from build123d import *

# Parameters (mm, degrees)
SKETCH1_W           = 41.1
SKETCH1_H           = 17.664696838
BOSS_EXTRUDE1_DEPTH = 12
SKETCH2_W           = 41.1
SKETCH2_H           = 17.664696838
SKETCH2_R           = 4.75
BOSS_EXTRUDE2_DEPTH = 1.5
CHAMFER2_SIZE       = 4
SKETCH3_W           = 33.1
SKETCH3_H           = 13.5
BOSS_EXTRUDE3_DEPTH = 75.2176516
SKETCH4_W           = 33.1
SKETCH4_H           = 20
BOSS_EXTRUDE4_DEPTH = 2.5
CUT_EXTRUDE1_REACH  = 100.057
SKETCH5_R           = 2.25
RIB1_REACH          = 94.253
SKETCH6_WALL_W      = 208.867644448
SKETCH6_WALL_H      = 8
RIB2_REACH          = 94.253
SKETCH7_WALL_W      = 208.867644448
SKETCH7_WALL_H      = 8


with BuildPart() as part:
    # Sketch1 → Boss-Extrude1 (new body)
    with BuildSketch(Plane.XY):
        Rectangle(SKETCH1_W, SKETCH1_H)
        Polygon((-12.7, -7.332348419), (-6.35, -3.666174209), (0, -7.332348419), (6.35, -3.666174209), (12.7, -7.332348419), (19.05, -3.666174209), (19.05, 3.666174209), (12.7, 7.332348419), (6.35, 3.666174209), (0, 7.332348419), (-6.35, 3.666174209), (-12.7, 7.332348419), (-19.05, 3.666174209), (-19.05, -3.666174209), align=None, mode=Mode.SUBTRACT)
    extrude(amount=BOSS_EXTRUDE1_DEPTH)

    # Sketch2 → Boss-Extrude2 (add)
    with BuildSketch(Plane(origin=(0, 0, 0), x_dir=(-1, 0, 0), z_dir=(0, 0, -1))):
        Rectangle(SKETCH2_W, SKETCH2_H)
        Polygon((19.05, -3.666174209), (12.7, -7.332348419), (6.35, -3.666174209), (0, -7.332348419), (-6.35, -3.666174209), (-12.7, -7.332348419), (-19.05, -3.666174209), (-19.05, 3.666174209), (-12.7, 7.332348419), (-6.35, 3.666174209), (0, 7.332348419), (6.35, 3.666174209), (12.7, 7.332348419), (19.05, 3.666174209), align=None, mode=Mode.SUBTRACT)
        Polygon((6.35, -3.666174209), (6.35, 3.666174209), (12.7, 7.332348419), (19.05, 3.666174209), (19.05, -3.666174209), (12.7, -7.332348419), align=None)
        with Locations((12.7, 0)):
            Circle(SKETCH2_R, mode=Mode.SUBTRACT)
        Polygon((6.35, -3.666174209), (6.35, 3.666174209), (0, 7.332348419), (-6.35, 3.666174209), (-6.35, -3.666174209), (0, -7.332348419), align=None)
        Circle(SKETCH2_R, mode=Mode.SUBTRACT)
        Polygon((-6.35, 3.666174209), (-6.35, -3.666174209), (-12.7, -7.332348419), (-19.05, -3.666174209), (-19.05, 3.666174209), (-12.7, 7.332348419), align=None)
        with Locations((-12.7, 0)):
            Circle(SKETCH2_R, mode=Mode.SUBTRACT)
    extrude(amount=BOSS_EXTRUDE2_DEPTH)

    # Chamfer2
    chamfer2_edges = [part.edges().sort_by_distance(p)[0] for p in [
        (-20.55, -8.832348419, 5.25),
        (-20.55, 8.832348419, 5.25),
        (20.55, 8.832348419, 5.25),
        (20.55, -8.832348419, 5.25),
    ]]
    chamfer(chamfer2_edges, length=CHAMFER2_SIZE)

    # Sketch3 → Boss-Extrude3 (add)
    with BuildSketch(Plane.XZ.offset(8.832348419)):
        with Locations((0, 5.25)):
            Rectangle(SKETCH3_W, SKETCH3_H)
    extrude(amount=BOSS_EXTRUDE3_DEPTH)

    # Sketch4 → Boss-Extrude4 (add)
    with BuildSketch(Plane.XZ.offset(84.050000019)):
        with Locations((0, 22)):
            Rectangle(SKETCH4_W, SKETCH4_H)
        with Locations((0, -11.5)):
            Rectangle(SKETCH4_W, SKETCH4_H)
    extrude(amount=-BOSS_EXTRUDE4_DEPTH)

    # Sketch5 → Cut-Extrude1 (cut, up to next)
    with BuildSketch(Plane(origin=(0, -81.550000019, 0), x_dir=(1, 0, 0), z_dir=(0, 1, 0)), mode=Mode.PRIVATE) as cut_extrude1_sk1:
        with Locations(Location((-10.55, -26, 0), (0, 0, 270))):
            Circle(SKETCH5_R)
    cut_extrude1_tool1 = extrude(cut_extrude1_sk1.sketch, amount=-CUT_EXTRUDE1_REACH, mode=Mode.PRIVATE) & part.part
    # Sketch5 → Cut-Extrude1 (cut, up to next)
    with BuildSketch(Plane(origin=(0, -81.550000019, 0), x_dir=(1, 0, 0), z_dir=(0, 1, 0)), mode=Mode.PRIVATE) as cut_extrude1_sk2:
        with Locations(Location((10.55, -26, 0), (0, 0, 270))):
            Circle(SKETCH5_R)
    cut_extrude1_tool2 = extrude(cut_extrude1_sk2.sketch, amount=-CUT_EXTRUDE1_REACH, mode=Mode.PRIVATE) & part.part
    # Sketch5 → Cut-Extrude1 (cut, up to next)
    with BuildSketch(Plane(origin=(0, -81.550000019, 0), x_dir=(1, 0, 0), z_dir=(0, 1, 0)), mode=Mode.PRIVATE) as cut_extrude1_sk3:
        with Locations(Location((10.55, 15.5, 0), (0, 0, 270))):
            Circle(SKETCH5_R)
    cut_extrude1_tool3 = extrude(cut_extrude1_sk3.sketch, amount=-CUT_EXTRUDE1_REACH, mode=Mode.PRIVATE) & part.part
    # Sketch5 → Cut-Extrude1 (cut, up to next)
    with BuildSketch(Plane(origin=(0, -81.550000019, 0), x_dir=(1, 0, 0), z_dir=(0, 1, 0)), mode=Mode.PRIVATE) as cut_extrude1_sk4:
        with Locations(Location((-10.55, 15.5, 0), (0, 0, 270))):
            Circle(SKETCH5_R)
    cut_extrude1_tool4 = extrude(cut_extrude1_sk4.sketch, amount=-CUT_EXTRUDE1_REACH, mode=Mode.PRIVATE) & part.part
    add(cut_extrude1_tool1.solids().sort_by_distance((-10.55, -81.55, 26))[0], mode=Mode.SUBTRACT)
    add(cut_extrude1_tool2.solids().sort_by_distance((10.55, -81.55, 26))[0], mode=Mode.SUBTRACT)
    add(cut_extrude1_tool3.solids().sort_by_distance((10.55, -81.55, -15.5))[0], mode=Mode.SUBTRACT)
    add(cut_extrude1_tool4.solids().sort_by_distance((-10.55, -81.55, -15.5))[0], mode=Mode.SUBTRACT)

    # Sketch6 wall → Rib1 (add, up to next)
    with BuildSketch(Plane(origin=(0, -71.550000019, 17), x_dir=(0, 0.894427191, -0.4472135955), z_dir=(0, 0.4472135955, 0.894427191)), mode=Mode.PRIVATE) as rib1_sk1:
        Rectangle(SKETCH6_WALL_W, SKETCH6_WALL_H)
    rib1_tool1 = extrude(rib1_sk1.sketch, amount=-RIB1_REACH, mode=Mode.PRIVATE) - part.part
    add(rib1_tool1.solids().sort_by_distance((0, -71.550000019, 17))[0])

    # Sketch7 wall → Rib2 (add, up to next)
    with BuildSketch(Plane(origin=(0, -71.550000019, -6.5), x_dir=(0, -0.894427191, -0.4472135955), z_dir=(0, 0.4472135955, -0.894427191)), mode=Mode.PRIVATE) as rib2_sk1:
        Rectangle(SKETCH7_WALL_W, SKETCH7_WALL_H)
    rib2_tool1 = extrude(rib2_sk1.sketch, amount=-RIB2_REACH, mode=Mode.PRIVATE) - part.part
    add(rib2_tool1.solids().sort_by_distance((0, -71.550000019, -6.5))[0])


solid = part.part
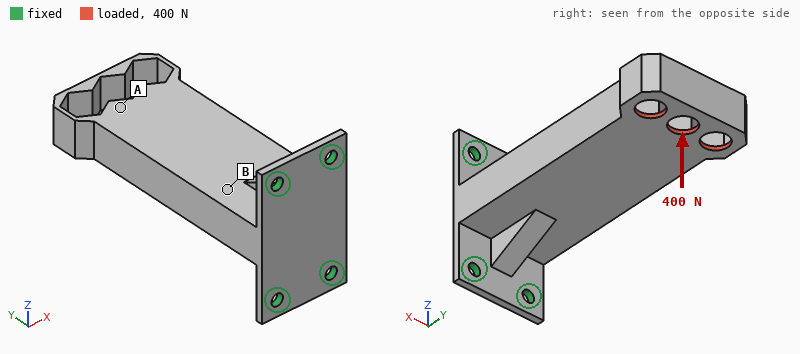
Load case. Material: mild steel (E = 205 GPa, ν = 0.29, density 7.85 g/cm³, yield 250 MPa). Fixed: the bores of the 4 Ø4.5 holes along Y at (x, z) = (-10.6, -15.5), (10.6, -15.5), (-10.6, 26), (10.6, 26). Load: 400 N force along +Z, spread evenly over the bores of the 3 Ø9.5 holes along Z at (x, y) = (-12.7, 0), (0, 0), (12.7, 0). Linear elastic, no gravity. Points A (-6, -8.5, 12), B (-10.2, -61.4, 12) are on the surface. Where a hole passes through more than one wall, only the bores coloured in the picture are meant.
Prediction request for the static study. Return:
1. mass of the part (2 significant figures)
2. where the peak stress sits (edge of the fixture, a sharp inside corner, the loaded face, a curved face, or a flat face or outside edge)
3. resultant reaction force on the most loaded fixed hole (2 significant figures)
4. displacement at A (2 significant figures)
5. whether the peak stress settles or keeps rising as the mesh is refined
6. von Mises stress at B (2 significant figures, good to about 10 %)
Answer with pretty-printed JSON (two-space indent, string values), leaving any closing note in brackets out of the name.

{
  "mass of the part": "330 g",
  "where the peak stress sits": "edge of the fixture",
  "resultant reaction force on the most loaded fixed hole": "500 N",
  "displacement at A": "0.079 mm",
  "whether the peak stress settles or keeps rising as the mesh is refined": "keeps rising",
  "von Mises stress at B": "21 MPa"
}
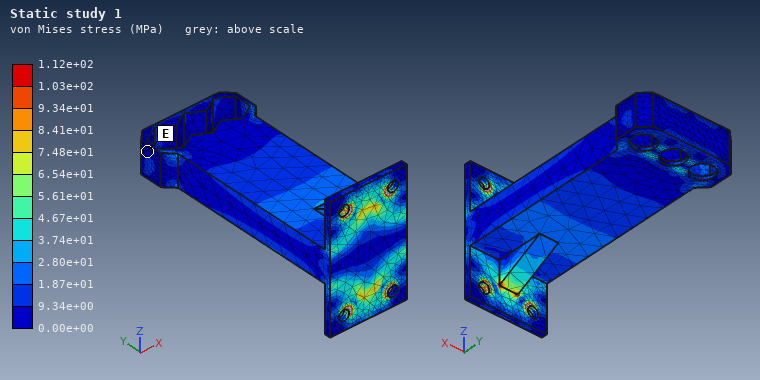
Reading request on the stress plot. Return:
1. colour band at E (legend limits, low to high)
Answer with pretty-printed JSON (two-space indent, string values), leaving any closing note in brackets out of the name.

{
  "colour band at E": "0.00e+00 to 9.34e+00 MPa"
}
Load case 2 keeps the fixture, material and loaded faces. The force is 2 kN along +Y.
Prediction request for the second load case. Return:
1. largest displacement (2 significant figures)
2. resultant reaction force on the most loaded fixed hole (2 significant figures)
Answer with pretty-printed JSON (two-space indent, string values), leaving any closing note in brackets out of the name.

{
  "largest displacement": "57 µm",
  "resultant reaction force on the most loaded fixed hole": "740 N"
}
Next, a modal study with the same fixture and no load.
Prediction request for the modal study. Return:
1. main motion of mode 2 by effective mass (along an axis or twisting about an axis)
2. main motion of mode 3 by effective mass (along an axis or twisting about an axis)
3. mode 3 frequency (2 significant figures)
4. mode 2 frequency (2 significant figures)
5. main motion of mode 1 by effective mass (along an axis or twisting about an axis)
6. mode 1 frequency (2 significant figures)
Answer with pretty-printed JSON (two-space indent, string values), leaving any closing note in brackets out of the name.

{
  "main motion of mode 2 by effective mass": "along Z",
  "main motion of mode 3 by effective mass": "along Y",
  "mode 3 frequency": "3700 Hz",
  "mode 2 frequency": "1100 Hz",
  "main motion of mode 1 by effective mass": "along X",
  "mode 1 frequency": "640 Hz"
}
